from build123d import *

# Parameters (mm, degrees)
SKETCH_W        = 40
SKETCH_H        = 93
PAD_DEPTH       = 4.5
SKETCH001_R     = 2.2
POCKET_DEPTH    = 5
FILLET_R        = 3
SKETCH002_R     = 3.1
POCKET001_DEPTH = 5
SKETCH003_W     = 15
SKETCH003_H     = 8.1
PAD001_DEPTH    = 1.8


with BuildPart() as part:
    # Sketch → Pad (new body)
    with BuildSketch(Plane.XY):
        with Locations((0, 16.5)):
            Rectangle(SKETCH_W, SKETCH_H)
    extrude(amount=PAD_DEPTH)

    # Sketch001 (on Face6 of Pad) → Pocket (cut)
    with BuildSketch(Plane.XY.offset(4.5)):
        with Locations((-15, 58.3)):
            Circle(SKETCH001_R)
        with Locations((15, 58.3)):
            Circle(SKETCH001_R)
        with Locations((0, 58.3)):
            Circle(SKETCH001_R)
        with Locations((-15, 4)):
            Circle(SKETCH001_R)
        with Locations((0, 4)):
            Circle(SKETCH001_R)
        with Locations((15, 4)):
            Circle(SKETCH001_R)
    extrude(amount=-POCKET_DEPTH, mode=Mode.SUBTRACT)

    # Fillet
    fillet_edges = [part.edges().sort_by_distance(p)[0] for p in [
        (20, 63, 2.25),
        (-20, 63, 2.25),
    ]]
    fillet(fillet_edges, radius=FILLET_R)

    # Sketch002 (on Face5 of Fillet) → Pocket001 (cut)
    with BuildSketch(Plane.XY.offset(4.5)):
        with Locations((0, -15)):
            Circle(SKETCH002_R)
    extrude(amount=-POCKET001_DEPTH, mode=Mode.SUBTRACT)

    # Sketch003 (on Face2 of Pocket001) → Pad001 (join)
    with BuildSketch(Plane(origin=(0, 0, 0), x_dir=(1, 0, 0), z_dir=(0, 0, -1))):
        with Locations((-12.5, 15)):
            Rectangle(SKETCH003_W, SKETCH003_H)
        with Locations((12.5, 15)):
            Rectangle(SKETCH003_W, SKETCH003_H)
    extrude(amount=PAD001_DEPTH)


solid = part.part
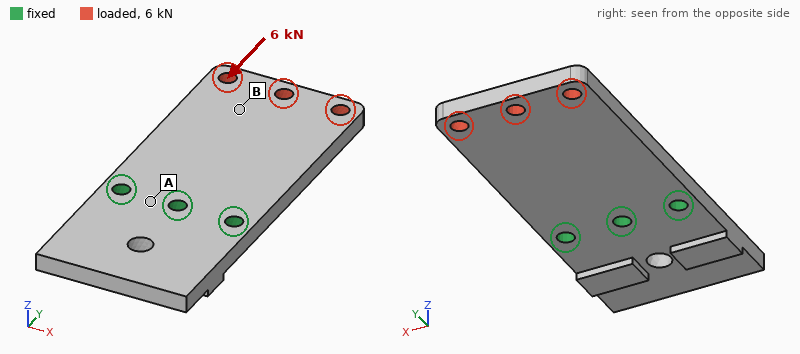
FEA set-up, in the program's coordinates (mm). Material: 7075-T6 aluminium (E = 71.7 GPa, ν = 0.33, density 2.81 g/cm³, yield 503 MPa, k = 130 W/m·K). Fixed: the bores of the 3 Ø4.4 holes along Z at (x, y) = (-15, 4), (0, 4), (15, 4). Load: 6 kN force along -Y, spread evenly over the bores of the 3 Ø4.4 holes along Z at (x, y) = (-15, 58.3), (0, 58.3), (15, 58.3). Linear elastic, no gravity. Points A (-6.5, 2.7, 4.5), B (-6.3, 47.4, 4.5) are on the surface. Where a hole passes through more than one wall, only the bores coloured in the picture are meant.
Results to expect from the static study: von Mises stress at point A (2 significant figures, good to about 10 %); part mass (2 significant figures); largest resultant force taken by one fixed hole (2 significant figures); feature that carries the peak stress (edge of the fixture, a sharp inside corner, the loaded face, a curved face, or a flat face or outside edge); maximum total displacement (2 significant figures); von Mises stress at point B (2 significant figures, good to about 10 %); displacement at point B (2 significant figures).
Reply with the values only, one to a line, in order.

12 MPa
47 g
2.0 kN
the loaded face
31 µm
31 MPa
20 µm
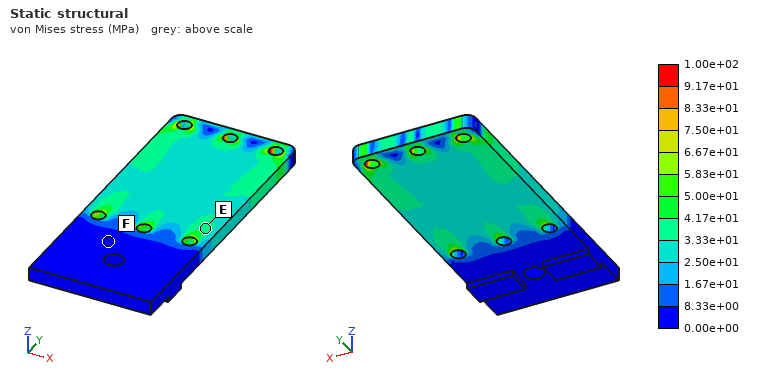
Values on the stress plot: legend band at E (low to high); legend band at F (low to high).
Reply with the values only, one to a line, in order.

3.33e+01 to 4.17e+01 MPa
0.00e+00 to 8.33e+00 MPa
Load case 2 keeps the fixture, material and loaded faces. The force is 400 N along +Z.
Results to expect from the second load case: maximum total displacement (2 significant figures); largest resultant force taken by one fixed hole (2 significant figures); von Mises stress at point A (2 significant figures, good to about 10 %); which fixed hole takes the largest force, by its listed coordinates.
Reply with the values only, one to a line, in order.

1.0 mm
360 N
41 MPa
(0, 4)
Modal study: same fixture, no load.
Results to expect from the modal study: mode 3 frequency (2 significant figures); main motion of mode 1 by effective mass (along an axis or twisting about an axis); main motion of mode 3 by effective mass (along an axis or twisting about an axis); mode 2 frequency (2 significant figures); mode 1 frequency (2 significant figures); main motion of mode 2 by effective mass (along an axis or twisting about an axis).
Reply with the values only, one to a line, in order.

3600 Hz
along Z
twisting about Y
3300 Hz
1100 Hz
along Z
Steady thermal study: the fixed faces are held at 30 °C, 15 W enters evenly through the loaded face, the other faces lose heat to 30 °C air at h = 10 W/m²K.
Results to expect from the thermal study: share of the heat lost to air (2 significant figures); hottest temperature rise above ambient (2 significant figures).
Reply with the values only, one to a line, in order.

6.4 %
35 K
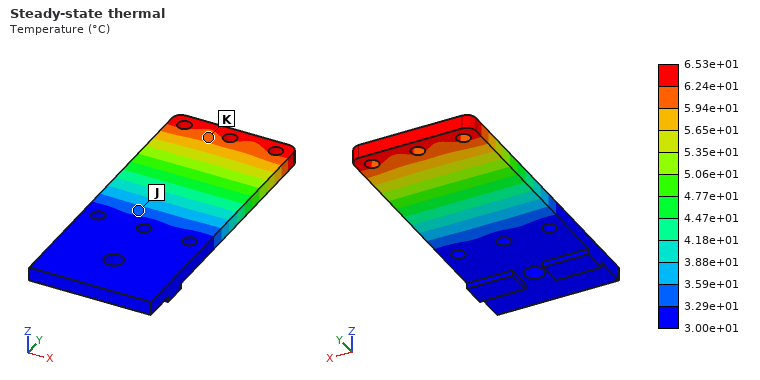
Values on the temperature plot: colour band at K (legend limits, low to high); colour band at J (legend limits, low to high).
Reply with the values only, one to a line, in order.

5.94e+01 to 6.24e+01 °C
3.29e+01 to 3.59e+01 °C
